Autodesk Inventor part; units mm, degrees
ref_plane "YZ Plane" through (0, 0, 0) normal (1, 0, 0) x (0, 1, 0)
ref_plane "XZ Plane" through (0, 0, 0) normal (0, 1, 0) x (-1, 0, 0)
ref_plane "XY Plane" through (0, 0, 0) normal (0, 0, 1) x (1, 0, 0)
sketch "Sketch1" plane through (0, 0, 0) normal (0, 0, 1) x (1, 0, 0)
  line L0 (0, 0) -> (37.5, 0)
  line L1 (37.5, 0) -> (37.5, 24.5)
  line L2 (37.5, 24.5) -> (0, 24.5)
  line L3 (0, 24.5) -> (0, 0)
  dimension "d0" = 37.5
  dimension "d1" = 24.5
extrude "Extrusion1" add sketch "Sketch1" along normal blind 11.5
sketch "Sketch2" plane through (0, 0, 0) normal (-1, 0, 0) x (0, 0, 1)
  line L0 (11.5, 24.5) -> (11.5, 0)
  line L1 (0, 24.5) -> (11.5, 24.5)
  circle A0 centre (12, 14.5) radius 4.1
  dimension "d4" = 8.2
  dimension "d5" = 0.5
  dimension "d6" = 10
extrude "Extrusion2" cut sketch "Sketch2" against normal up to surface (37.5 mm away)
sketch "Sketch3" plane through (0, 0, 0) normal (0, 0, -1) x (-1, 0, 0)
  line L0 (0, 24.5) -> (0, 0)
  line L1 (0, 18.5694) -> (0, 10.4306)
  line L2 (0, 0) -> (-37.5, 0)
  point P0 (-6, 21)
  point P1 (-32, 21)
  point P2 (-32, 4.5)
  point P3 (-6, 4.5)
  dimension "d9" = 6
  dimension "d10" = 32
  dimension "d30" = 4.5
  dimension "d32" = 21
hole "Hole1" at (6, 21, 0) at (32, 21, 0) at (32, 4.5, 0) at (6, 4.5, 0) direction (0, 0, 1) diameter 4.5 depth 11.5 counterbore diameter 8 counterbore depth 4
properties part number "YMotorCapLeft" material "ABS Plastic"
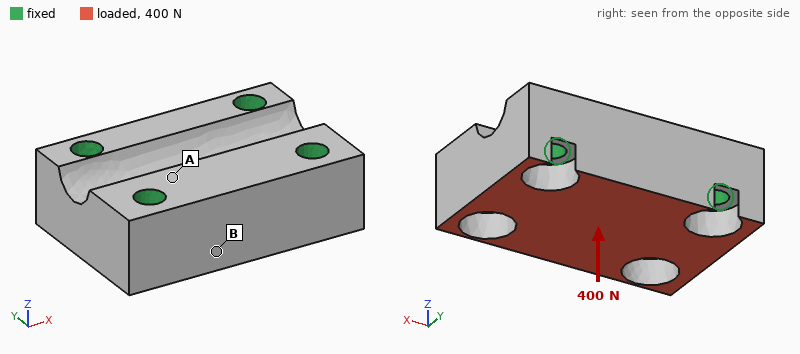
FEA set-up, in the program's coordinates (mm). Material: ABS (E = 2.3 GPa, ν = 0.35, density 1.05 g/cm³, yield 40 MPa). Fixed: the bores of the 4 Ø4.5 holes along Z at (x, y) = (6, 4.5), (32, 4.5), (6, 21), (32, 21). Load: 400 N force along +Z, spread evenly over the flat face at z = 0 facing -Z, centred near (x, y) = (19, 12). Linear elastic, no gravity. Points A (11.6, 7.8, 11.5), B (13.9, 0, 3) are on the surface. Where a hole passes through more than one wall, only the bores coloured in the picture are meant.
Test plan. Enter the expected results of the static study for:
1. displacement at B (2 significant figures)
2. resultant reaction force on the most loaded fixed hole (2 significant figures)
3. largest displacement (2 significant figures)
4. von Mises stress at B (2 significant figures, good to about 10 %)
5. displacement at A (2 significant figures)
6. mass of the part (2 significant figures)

7.8 µm
120 N
10 µm
0.77 MPa
6.2 µm
8.9 g
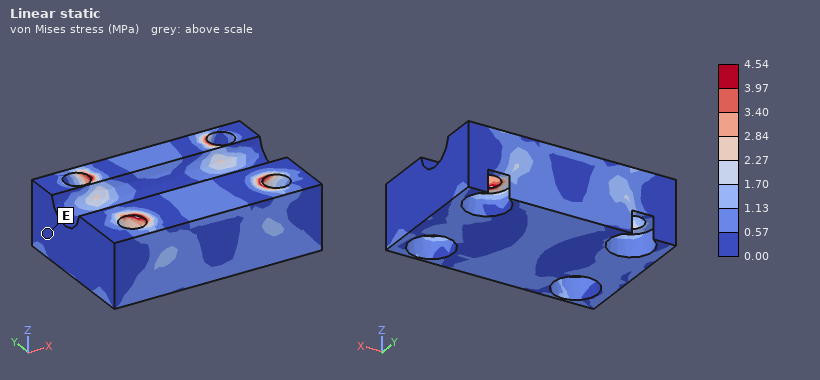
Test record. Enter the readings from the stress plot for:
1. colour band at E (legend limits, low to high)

0.00 to 0.57 MPa
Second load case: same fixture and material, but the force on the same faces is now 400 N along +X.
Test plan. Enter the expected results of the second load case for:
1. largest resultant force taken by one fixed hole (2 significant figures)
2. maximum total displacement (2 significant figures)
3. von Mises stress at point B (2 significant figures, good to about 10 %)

120 N
23 µm
1.2 MPa
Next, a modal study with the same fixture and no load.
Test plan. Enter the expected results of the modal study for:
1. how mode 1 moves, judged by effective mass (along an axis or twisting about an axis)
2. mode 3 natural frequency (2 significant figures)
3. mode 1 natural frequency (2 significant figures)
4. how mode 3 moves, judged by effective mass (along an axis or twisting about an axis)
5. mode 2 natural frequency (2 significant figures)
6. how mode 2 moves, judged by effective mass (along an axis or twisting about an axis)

along Z
15 kHz
12 kHz
along Y
14 kHz
along Y
